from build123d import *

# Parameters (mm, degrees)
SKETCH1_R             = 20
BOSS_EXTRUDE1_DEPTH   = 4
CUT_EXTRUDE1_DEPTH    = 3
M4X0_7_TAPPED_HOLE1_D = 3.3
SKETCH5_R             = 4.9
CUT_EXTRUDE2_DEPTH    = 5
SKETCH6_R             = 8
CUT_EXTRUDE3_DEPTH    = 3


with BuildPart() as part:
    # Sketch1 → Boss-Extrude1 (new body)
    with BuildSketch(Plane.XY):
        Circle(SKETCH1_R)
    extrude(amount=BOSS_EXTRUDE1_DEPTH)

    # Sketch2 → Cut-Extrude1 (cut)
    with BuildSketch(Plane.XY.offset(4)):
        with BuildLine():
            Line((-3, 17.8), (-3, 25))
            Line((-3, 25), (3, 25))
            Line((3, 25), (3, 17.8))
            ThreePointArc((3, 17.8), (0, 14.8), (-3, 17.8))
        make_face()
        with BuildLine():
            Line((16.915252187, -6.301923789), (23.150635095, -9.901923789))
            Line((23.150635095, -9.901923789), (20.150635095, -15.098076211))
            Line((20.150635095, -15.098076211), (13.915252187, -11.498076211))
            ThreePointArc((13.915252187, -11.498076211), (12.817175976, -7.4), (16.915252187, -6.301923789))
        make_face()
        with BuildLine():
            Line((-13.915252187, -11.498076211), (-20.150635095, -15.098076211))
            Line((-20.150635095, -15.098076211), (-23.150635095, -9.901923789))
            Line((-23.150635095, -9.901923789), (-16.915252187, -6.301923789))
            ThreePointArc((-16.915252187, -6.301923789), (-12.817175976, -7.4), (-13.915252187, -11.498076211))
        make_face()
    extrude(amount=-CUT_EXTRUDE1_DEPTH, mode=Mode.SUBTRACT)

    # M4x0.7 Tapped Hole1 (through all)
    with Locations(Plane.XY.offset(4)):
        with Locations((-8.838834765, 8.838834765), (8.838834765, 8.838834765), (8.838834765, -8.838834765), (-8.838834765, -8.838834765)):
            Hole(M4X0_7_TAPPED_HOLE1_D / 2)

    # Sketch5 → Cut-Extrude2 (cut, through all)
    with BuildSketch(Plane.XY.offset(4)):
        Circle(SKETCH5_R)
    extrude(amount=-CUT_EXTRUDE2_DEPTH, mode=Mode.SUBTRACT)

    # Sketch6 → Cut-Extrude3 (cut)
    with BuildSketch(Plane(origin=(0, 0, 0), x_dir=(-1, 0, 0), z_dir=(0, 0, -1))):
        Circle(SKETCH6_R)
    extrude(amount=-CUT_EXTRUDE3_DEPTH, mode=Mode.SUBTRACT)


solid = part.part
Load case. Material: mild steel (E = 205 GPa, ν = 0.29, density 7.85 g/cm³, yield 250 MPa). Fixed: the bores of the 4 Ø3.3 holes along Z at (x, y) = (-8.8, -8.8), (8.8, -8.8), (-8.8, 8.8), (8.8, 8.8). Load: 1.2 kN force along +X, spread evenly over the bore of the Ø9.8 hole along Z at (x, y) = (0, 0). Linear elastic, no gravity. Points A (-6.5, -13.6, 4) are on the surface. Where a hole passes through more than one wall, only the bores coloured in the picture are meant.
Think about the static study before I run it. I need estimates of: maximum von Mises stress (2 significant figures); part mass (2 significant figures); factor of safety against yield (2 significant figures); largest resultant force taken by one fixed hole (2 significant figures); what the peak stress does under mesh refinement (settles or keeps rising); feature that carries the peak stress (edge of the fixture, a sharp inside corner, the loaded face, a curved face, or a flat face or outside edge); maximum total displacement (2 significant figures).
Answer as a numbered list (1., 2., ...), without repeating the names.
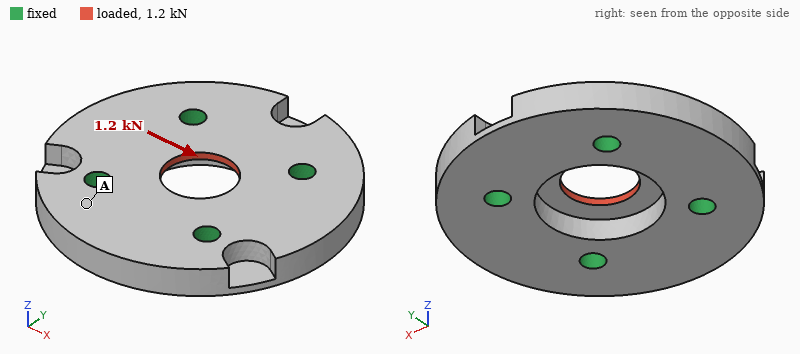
1. 69 MPa
2. 31 g
3. 3.6
4. 310 N
5. settles
6. the loaded face
7. 1.8 µm
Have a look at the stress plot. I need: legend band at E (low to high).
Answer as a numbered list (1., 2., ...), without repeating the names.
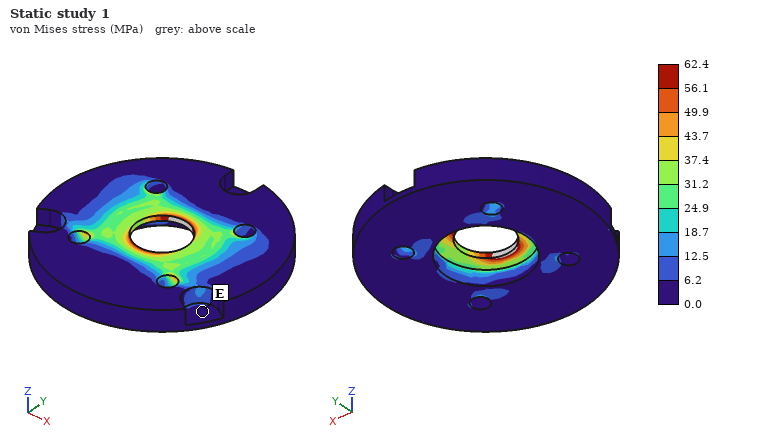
1. 0.0 to 6.2 MPa
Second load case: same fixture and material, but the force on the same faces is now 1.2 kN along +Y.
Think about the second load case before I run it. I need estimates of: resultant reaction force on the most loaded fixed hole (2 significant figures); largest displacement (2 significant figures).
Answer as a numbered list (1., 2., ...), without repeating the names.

1. 310 N
2. 1.8 µm
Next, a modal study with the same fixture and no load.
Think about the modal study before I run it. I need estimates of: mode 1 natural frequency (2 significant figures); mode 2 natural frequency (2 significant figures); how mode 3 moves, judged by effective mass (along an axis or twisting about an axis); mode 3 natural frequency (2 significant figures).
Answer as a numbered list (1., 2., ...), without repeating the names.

1. 25 kHz
2. 25 kHz
3. along Z
4. 27 kHz
